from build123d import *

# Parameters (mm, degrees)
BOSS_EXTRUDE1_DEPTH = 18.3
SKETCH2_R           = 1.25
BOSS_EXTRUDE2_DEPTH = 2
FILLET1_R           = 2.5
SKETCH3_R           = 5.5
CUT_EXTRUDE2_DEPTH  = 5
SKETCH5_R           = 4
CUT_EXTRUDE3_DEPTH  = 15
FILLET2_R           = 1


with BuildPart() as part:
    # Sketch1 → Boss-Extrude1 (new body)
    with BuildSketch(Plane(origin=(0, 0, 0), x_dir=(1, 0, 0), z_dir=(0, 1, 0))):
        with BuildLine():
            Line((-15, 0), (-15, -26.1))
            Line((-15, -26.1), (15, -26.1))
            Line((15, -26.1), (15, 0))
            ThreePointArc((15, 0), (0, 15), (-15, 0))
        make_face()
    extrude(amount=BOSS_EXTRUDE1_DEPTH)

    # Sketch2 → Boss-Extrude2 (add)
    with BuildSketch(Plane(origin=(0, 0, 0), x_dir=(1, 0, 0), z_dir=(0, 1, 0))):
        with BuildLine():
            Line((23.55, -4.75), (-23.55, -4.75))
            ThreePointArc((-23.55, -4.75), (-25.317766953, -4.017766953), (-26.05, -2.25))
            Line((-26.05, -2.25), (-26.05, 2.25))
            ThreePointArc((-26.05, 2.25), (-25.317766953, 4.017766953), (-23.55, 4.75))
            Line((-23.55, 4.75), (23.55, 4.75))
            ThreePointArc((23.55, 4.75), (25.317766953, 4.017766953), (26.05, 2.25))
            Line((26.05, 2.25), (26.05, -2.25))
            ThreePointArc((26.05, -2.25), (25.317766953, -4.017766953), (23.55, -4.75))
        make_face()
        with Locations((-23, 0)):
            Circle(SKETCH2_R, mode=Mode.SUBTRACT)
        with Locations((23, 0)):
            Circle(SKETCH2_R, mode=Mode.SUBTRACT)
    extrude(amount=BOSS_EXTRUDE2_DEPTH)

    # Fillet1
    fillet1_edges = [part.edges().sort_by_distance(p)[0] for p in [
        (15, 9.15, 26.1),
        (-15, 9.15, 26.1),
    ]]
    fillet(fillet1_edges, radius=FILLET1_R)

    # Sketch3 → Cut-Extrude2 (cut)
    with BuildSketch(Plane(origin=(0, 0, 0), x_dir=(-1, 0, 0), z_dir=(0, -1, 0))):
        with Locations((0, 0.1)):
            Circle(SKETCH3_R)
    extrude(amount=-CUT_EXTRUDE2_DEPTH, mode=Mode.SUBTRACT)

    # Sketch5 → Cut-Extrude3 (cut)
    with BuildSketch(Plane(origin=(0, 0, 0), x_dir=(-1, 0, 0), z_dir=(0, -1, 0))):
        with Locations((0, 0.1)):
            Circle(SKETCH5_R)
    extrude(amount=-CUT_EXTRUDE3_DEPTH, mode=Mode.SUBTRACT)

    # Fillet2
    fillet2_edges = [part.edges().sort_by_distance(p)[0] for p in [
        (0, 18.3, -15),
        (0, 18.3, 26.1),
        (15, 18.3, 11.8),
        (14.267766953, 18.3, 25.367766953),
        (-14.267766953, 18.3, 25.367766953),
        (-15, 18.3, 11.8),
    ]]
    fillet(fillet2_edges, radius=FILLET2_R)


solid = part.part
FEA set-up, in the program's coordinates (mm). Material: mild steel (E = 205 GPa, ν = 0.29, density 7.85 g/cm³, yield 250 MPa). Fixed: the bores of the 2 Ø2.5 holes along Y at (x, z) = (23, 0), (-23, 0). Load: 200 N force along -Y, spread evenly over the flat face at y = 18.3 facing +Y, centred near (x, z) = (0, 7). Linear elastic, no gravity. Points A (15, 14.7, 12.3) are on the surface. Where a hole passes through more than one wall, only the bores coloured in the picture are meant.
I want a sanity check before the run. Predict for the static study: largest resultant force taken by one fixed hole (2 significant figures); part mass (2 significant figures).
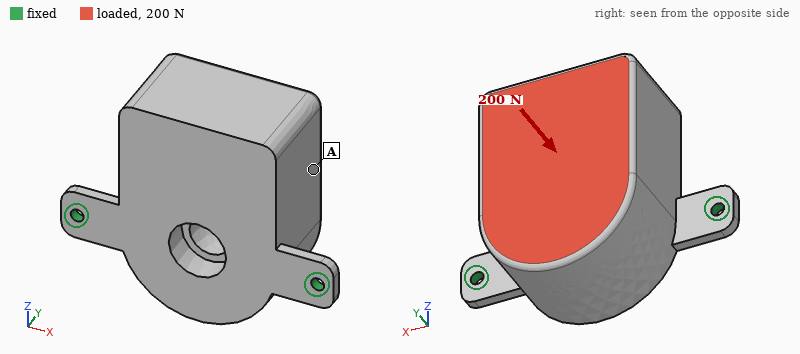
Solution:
110 N
160 g
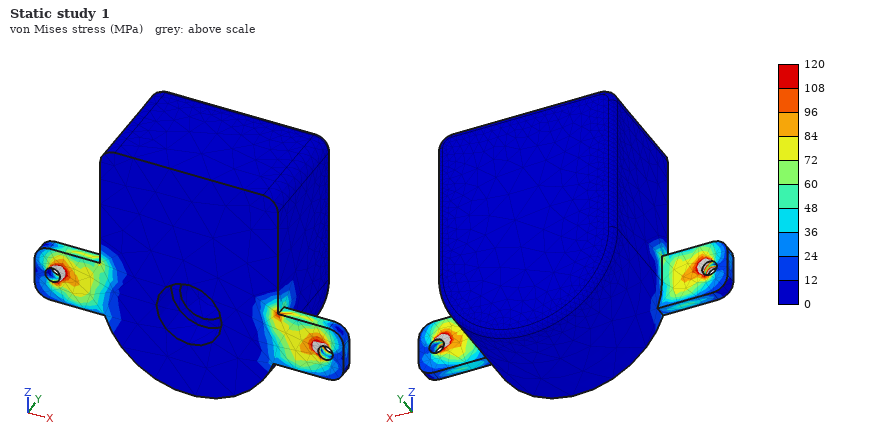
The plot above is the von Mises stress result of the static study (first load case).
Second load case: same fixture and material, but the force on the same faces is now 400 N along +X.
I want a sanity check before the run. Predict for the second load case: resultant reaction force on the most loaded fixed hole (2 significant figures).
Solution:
280 N
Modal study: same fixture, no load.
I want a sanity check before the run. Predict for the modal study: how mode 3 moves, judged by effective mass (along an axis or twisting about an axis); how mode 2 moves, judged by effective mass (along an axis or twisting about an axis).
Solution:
along X
along Y
